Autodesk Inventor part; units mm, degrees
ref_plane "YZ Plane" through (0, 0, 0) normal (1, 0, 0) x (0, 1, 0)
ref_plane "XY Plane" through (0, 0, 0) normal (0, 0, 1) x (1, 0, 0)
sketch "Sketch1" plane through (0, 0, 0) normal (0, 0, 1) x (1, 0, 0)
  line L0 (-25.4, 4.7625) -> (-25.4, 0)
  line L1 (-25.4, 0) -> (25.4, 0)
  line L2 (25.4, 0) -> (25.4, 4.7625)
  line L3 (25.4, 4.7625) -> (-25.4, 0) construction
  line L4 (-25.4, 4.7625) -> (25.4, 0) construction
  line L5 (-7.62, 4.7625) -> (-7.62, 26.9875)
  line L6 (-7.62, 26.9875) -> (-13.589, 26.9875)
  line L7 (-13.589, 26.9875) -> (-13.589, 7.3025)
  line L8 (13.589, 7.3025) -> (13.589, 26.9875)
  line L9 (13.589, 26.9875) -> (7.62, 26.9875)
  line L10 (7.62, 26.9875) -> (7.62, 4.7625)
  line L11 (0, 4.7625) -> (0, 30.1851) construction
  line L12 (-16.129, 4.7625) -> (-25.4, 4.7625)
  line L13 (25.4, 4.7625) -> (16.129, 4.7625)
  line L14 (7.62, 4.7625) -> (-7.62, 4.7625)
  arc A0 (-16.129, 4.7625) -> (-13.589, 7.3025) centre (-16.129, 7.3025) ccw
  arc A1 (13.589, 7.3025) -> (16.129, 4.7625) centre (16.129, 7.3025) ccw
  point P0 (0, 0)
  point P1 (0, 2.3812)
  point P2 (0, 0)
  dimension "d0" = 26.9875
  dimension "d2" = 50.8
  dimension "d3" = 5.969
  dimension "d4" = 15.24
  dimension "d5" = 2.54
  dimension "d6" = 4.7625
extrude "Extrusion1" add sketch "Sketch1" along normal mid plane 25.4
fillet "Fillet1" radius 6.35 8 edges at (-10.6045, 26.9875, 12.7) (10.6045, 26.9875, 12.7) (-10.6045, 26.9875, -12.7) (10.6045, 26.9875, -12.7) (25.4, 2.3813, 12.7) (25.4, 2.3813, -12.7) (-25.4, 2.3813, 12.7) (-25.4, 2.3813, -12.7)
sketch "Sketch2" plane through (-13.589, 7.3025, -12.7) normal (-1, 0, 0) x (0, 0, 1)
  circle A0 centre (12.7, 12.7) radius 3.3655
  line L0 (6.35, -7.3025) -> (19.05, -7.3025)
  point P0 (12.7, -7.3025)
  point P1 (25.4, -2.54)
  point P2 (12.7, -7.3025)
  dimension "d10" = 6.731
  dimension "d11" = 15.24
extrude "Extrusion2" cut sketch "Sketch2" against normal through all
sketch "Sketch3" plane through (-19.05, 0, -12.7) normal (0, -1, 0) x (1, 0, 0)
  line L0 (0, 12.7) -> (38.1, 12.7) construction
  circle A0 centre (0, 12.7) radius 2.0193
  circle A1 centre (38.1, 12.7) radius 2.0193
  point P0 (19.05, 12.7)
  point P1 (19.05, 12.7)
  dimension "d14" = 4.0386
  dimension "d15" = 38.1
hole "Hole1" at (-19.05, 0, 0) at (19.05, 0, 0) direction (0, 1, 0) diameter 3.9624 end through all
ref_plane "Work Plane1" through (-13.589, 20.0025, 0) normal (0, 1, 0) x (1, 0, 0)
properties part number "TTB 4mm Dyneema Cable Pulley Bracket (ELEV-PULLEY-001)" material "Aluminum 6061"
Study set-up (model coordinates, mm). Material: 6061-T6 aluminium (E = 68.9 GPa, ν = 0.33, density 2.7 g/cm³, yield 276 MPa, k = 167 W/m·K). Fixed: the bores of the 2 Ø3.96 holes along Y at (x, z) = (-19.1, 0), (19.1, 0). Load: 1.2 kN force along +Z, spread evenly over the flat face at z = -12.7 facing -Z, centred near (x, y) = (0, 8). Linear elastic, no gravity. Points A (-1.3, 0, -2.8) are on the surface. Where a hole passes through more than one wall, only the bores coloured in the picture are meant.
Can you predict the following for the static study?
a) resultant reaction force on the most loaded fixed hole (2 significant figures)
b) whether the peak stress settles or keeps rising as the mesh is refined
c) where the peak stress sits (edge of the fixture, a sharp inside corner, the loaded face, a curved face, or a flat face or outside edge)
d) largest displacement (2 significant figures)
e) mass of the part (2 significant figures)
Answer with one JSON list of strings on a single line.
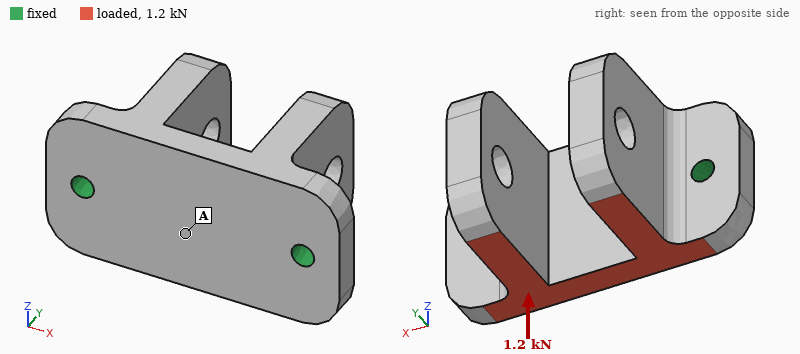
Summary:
["600 N", "keeps rising", "edge of the fixture", "28 µm", "33 g"]
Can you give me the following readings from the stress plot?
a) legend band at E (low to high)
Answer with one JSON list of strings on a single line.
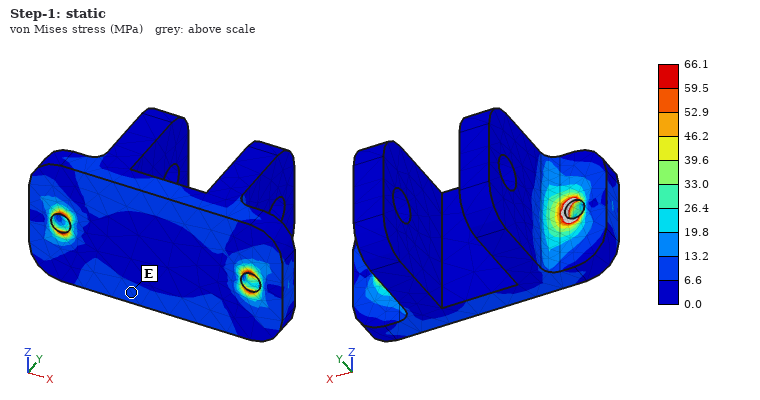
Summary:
["6.6 to 13.2 MPa"]
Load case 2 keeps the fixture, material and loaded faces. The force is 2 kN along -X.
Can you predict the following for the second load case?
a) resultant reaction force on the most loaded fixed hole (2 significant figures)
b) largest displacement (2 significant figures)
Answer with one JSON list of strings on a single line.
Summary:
["1.2 kN", "35 µm"]
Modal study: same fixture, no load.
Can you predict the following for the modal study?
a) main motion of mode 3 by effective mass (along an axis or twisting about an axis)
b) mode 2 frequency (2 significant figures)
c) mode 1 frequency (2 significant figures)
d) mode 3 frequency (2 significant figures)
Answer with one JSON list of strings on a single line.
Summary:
["along X", "5600 Hz", "5600 Hz", "8300 Hz"]
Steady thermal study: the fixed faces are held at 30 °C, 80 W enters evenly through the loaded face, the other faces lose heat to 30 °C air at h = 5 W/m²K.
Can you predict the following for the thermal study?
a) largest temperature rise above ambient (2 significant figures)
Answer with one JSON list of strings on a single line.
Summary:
["34 K"]
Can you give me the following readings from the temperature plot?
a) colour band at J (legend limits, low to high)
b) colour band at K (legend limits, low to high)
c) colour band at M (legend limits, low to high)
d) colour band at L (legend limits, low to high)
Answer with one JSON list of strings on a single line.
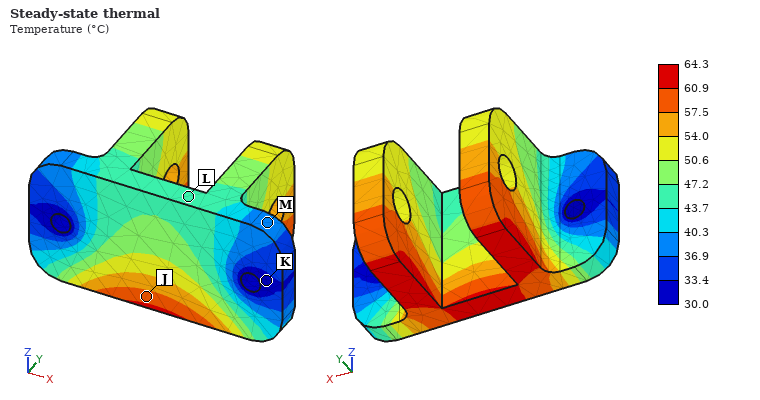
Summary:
["57.5 to 60.9 °C", "30.0 to 33.4 °C", "36.9 to 40.3 °C", "43.7 to 47.2 °C"]
